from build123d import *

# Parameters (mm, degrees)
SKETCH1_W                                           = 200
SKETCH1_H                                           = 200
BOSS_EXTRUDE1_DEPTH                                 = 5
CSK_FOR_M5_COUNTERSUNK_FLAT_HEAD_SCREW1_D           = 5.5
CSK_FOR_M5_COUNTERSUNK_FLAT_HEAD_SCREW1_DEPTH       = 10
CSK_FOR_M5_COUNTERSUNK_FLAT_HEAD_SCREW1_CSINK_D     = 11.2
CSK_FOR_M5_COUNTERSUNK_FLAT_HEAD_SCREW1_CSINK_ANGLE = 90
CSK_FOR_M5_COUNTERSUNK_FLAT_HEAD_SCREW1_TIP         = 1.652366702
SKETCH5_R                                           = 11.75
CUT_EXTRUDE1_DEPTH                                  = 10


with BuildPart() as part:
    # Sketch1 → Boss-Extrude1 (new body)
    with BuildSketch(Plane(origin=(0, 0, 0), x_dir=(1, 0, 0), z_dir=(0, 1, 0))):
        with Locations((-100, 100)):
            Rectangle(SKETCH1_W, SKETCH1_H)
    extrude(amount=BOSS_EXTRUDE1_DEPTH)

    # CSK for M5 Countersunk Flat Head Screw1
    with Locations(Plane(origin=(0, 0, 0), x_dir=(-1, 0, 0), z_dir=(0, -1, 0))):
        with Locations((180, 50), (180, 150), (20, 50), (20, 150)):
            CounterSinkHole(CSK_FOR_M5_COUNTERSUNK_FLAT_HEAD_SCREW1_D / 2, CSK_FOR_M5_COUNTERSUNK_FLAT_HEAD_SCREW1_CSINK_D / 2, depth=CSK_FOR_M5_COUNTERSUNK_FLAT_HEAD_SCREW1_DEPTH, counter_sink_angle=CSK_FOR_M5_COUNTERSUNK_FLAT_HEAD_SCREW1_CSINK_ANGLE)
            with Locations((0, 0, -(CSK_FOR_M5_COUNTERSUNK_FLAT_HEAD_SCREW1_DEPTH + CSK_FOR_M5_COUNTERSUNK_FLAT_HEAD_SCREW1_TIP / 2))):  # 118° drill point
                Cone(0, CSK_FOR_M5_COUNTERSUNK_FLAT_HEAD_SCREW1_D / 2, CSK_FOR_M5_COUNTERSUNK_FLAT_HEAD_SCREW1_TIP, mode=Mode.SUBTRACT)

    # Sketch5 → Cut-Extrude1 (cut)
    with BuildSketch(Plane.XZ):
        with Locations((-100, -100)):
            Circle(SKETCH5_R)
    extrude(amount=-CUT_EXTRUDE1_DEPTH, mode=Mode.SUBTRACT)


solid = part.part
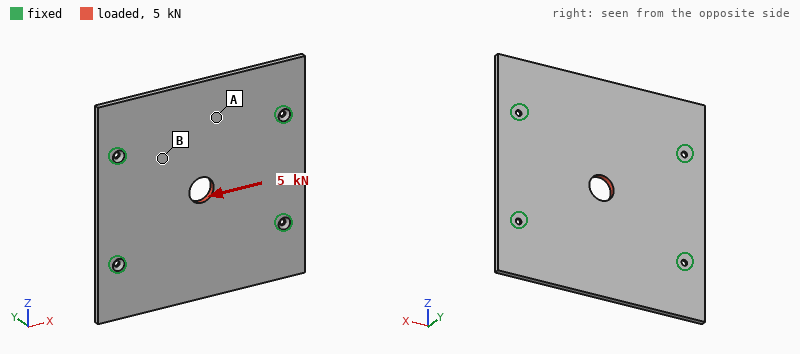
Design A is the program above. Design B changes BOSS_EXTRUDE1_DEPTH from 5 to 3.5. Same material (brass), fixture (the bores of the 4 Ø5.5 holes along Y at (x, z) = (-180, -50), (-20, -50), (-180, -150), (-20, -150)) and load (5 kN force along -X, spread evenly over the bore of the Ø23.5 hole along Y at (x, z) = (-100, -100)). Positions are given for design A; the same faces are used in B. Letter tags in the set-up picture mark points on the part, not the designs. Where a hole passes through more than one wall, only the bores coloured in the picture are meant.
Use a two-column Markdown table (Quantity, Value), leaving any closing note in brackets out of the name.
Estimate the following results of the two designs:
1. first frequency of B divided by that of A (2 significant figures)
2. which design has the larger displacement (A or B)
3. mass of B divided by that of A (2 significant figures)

| Quantity | Value |
|---|---|
| first frequency of B divided by that of A | 0.69 |
| which design has the larger displacement | B |
| mass of B divided by that of A | 0.70 |
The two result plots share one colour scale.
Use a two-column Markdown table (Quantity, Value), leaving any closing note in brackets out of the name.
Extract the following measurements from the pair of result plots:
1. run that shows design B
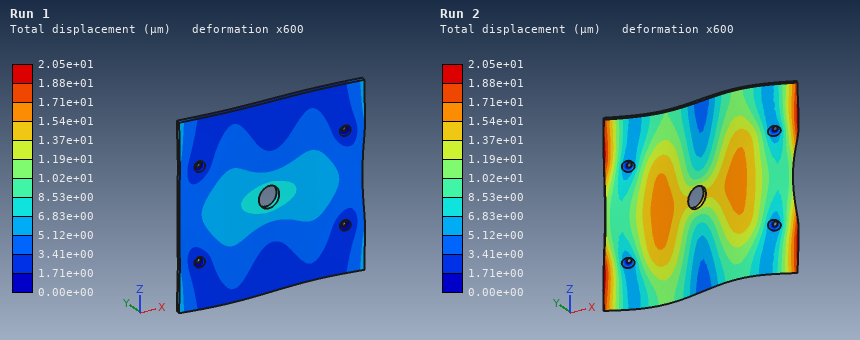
| Quantity | Value |
|---|---|
| run that shows design B | Run 2 |
